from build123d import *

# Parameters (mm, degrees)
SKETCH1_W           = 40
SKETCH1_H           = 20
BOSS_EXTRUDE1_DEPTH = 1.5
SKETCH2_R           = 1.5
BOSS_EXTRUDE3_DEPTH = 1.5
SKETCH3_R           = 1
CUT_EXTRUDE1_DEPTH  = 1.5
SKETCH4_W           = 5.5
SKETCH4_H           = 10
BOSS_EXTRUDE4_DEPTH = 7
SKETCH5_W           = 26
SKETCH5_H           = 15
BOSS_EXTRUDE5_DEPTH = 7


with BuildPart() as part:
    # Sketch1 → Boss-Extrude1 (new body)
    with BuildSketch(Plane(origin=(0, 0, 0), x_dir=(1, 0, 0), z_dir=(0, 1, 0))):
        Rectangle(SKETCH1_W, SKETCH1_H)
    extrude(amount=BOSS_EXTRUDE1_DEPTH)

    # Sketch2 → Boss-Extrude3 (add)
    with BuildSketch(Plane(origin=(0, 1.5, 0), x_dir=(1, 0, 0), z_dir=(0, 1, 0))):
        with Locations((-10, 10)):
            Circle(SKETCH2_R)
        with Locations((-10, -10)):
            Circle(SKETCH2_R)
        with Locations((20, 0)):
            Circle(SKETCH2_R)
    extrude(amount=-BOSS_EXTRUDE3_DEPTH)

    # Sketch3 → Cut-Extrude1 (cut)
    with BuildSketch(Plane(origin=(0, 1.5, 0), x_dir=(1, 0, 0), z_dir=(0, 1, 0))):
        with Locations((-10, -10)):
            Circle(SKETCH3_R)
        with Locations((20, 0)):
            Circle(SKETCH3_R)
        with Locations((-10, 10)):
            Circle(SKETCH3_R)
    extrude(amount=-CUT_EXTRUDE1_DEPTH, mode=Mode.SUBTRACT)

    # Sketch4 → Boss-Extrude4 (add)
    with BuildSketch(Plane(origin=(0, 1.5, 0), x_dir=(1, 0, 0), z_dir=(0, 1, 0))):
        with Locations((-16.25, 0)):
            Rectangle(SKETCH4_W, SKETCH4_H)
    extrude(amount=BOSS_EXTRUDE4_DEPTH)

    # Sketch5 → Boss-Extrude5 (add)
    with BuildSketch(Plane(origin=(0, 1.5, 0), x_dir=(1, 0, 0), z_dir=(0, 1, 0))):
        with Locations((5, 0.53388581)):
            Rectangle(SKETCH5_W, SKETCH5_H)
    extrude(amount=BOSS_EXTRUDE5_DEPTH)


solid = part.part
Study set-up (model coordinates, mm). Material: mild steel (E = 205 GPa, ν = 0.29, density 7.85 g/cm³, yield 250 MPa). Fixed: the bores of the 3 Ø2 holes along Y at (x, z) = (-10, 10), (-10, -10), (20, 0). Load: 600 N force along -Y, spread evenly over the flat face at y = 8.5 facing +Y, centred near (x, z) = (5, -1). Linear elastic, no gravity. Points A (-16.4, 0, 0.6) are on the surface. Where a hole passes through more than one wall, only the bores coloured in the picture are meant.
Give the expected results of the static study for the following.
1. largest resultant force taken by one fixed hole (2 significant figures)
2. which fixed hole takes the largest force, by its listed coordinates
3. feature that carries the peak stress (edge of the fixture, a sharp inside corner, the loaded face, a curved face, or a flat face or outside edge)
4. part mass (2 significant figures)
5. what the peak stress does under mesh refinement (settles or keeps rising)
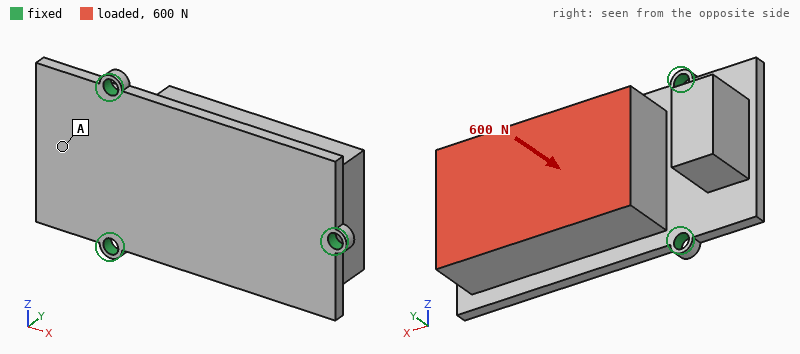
350 N
(20, 0)
edge of the fixture
34 g
keeps rising
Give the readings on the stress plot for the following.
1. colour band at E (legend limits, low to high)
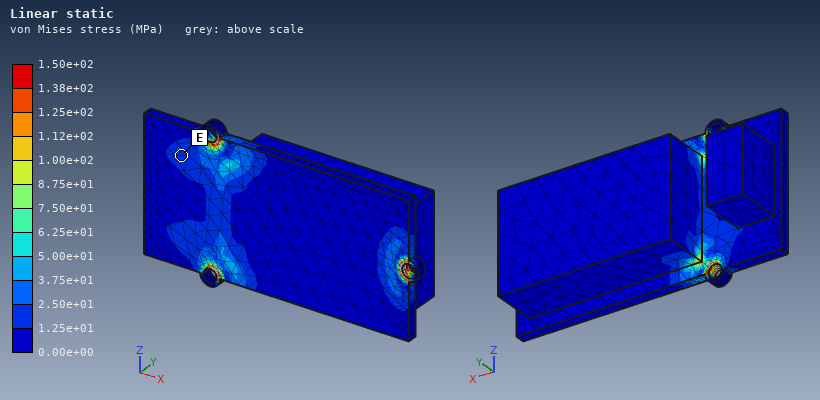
1.25e+01 to 2.50e+01 MPa
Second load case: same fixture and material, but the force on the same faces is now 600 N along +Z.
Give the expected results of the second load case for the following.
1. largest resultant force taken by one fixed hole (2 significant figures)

370 N
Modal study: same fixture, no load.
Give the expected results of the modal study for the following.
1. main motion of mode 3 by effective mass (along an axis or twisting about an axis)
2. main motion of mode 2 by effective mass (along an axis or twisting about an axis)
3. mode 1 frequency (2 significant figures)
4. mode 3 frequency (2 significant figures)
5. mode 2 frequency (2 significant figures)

along Y
along Z
5400 Hz
12 kHz
10 kHz
